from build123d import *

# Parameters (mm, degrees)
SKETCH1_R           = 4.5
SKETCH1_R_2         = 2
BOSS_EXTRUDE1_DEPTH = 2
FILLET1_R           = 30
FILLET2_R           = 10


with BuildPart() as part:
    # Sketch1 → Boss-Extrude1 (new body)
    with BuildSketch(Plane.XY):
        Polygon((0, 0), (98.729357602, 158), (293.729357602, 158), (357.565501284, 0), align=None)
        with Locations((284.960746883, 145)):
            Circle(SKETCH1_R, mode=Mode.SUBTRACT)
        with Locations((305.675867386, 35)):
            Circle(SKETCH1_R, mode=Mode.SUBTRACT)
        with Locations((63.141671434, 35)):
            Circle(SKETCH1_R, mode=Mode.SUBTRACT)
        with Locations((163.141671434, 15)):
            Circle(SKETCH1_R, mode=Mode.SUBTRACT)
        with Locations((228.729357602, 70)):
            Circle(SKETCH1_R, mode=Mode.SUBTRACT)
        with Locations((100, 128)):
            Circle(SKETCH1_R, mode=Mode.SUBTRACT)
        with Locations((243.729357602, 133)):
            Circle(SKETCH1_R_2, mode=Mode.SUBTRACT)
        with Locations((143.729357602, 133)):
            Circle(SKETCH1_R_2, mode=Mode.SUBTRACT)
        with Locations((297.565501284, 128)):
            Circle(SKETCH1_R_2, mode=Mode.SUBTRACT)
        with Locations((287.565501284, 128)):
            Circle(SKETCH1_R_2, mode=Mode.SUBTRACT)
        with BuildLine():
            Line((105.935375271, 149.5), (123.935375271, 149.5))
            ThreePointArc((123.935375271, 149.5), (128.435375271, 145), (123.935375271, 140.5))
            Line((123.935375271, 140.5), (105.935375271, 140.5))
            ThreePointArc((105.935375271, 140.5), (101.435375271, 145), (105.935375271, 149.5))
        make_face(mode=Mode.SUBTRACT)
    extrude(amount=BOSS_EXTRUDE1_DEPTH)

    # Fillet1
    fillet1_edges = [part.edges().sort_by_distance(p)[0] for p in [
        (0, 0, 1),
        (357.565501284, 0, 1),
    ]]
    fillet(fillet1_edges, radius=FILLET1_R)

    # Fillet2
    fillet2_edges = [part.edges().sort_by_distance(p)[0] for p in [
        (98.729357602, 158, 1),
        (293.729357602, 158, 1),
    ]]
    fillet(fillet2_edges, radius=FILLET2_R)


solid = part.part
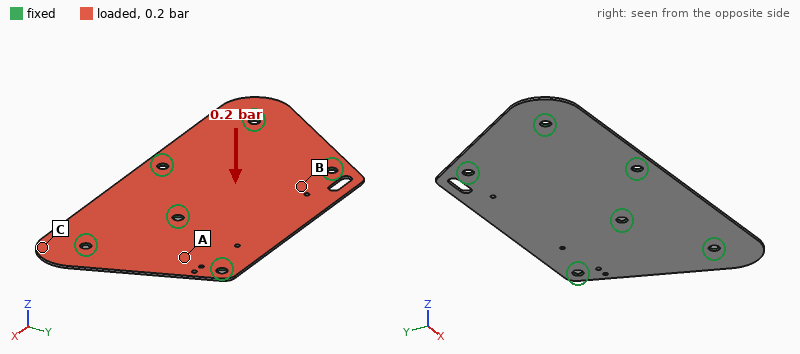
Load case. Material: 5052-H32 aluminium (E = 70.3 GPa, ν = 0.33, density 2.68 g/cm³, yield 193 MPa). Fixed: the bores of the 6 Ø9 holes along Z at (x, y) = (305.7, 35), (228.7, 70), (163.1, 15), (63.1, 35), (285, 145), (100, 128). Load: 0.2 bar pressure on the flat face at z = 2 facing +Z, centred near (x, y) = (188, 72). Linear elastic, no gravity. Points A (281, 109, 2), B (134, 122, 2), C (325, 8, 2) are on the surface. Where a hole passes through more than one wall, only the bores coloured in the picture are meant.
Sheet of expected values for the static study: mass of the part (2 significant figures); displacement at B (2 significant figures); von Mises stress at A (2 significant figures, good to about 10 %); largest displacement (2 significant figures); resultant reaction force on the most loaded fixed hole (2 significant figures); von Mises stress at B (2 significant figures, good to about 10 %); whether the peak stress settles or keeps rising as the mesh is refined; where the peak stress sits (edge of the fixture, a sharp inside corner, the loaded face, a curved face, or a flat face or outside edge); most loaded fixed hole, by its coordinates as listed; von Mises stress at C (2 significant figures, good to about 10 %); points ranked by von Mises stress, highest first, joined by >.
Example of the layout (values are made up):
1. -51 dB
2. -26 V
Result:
1. 220 g
2. 0.32 mm
3. 14 MPa
4. 1.0 mm
5. 210 N
6. 22 MPa
7. keeps rising
8. edge of the fixture
9. (228.7, 70)
10. 6.9 MPa
11. B > A > C
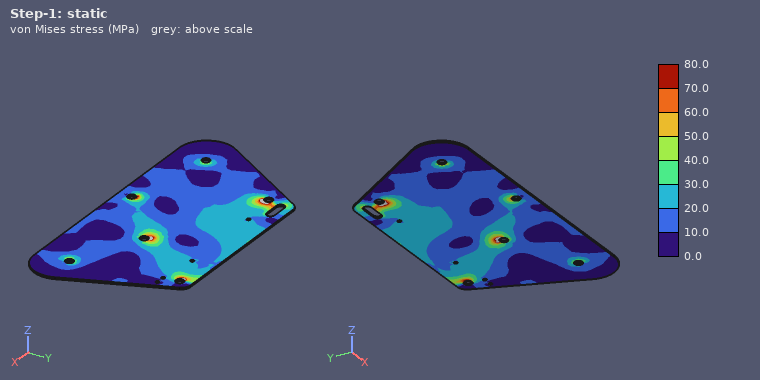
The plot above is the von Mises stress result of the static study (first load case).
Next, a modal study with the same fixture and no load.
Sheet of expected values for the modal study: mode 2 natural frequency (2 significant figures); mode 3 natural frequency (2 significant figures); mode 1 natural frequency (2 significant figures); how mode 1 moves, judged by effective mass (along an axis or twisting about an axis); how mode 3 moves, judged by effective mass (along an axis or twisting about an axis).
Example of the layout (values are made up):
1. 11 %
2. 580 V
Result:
1. 700 Hz
2. 760 Hz
3. 410 Hz
4. along Z
5. along Z
